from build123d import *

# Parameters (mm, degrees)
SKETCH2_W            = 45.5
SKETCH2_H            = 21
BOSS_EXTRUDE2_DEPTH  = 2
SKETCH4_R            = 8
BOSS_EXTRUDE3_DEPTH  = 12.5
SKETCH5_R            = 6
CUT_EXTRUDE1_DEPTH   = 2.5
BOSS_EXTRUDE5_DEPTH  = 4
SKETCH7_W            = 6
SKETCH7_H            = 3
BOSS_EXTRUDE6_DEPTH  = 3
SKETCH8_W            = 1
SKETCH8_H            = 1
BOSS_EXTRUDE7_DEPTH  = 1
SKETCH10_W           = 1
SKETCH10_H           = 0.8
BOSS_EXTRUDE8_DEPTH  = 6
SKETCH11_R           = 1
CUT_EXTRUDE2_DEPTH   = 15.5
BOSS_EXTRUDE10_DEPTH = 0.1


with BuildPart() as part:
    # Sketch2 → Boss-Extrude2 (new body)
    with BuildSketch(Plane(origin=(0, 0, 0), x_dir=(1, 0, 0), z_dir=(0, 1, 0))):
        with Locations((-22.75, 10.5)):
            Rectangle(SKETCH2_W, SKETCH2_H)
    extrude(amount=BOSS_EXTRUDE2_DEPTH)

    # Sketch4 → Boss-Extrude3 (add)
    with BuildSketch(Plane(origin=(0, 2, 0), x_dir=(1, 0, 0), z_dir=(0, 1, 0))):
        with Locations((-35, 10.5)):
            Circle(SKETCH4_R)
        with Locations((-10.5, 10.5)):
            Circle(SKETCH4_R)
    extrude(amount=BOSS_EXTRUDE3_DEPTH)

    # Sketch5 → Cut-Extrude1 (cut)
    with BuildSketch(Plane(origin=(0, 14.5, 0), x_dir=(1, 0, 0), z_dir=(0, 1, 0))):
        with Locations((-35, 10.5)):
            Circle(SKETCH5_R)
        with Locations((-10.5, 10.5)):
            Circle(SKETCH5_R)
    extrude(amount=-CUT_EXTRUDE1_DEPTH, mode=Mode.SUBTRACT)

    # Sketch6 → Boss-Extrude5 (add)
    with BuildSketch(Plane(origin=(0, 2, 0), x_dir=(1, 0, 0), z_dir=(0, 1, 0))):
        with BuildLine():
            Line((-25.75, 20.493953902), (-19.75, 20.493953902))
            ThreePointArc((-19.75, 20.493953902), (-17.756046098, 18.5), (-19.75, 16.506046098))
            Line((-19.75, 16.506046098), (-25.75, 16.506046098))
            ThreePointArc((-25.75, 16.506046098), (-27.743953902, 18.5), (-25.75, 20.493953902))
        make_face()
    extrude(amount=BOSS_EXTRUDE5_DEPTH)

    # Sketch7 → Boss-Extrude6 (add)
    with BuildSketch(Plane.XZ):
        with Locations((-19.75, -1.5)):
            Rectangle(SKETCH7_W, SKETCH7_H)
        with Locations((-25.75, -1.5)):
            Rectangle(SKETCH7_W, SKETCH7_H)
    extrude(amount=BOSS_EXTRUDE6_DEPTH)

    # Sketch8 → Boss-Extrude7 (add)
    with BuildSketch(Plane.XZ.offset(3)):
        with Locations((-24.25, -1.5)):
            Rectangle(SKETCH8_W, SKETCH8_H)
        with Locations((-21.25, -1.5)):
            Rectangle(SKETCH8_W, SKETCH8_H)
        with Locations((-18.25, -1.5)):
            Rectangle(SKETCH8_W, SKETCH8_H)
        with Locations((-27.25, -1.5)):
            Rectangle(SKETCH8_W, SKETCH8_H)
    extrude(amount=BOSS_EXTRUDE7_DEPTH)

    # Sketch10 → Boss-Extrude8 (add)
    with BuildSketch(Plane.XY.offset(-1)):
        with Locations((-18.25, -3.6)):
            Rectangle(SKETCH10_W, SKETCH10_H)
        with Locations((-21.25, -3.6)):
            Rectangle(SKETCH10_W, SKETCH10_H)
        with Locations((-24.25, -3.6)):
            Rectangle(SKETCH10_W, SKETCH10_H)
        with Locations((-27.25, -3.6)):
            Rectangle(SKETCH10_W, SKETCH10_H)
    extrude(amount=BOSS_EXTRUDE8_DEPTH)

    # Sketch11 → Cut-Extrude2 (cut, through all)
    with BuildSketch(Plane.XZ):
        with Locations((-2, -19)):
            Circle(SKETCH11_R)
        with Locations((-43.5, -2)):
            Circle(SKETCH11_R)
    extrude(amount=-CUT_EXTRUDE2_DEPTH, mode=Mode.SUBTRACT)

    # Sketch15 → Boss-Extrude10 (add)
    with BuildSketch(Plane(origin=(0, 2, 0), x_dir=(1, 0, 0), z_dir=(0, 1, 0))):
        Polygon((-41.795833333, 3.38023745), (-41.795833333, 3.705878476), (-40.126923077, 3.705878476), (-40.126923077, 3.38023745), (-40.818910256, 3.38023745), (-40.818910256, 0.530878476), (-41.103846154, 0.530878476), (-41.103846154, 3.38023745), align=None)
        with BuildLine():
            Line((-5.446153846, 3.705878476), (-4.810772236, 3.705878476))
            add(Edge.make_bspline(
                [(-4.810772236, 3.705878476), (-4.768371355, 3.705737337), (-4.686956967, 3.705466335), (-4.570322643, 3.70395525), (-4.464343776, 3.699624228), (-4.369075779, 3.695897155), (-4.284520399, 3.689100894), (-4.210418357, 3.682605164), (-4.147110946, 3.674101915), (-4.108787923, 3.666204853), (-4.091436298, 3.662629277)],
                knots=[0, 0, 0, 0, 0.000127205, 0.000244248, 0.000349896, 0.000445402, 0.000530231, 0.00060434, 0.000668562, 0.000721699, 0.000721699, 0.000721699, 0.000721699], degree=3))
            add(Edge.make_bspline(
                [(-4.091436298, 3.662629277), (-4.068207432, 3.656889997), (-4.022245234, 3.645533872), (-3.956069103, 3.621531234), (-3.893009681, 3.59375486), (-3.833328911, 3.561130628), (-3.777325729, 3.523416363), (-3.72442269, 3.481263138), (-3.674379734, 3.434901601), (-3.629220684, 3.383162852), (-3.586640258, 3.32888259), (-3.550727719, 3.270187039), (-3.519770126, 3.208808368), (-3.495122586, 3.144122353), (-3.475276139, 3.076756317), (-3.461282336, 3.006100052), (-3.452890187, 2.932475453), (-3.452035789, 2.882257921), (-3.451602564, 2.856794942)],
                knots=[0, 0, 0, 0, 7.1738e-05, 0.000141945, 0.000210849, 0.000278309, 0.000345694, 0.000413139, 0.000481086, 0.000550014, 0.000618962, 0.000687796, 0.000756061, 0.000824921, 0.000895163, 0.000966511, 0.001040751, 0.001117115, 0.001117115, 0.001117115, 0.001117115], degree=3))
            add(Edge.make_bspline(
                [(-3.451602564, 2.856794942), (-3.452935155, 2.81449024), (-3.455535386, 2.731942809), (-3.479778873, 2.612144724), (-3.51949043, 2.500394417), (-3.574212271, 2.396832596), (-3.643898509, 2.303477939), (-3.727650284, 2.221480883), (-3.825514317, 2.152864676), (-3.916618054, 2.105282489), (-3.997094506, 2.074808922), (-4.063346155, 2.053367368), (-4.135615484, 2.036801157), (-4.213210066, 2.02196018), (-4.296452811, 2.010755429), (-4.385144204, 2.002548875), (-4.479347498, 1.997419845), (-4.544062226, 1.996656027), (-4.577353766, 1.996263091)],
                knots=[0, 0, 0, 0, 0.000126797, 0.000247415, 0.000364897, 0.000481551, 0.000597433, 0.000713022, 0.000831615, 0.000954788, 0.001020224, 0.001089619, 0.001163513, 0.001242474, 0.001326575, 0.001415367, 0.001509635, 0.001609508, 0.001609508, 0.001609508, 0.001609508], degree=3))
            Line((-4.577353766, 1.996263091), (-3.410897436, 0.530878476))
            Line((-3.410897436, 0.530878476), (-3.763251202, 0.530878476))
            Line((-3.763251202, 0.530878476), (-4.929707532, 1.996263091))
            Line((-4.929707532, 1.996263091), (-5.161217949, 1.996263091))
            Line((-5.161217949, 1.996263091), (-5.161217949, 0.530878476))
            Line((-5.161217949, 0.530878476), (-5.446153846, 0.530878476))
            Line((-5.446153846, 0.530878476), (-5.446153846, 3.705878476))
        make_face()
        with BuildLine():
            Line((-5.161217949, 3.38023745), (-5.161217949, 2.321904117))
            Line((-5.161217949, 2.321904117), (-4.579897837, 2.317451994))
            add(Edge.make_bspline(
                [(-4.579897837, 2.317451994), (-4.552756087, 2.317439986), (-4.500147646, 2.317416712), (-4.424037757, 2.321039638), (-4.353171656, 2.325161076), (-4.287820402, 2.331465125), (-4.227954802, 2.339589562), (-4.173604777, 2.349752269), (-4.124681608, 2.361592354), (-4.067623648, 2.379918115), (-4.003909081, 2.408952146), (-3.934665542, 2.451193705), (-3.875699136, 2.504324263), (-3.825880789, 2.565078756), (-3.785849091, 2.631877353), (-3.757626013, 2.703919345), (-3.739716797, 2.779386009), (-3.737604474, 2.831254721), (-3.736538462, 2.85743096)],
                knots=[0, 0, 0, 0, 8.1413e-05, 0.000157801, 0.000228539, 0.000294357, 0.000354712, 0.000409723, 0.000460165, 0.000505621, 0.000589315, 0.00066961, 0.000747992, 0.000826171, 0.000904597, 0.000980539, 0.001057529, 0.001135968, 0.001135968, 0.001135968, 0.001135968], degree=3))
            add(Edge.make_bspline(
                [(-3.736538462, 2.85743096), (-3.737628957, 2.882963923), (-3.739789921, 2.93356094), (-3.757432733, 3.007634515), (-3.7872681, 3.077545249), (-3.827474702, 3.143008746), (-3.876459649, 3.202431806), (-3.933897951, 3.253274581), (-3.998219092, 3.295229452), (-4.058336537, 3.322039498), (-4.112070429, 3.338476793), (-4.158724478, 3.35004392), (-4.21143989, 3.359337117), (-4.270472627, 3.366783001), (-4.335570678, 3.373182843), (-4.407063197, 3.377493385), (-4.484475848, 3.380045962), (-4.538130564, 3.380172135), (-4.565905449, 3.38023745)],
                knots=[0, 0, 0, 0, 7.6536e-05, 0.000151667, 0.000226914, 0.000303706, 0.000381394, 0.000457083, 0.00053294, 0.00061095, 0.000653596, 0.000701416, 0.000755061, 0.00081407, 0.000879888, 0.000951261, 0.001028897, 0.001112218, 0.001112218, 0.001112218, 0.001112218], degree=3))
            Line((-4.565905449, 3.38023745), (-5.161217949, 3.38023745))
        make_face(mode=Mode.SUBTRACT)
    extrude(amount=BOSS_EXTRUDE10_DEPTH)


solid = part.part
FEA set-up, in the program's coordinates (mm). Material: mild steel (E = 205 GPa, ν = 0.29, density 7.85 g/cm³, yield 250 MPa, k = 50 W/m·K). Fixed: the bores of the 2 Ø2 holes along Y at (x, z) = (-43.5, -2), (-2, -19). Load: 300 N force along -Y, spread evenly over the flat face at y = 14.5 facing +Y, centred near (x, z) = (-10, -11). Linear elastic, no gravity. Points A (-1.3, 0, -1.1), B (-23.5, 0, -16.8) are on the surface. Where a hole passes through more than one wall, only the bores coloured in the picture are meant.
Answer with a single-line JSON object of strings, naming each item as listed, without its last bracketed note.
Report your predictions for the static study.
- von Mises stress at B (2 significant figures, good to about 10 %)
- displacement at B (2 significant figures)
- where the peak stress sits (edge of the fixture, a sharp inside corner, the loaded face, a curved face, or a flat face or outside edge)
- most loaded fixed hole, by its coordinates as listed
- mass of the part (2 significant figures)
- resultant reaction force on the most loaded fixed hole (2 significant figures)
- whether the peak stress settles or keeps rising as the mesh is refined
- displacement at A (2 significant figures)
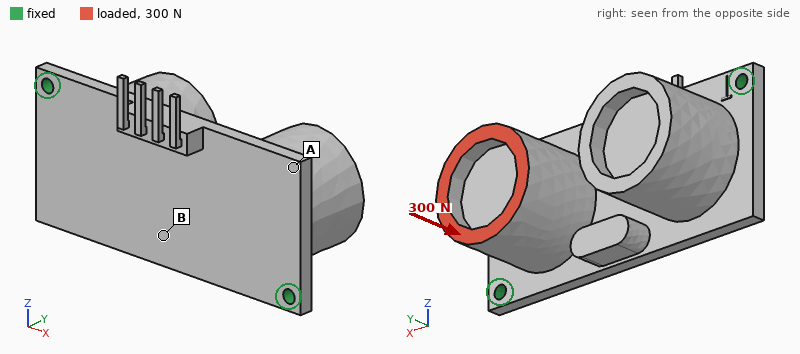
{"von Mises stress at B": "27 MPa", "displacement at B": "11 µm", "where the peak stress sits": "edge of the fixture", "most loaded fixed hole, by its coordinates as listed": "(-2, -19)", "mass of the part": "52 g", "resultant reaction force on the most loaded fixed hole": "240 N", "whether the peak stress settles or keeps rising as the mesh is refined": "keeps rising", "displacement at A": "39 µm"}
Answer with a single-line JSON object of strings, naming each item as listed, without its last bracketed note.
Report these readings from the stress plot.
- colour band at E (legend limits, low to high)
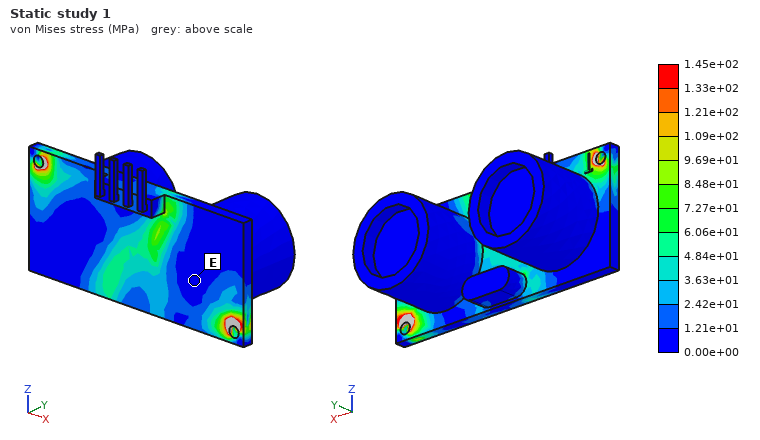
{"colour band at E": "0.00e+00 to 1.21e+01 MPa"}
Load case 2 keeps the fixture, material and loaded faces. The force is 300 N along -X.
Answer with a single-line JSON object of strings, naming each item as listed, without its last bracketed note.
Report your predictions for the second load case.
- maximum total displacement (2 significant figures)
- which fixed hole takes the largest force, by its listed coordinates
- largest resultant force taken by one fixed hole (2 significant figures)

{"maximum total displacement": "52 µm", "which fixed hole takes the largest force, by its listed coordinates": "(-2, -19)", "largest resultant force taken by one fixed hole": "190 N"}
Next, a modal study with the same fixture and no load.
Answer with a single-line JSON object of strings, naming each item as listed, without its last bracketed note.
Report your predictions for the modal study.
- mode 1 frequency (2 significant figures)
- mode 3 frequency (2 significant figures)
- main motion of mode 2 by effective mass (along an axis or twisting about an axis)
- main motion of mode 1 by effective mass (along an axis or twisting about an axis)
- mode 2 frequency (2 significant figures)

{"mode 1 frequency": "2200 Hz", "mode 3 frequency": "4900 Hz", "main motion of mode 2 by effective mass": "along Y", "main motion of mode 1 by effective mass": "along Z", "mode 2 frequency": "2600 Hz"}
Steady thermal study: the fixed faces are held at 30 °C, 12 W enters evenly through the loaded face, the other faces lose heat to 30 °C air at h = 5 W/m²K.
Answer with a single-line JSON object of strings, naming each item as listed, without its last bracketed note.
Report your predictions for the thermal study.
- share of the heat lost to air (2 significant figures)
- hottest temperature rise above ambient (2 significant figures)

{"share of the heat lost to air": "6.6 %", "hottest temperature rise above ambient": "75 K"}
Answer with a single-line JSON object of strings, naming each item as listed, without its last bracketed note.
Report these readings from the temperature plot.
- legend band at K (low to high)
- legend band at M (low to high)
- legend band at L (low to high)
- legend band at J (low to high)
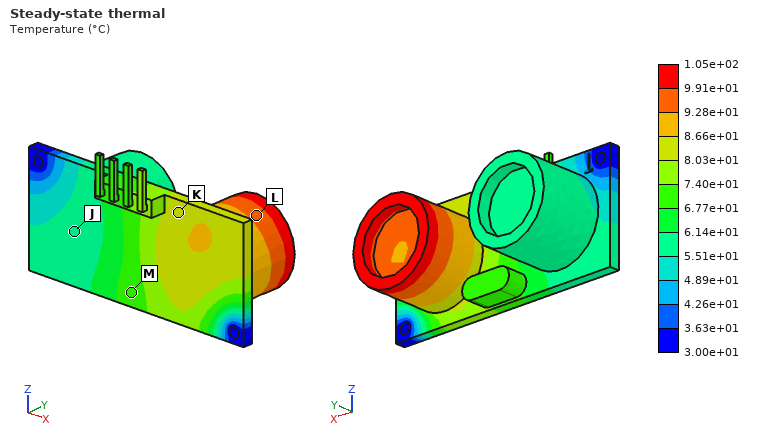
{"legend band at K": "8.03e+01 to 8.66e+01 °C", "legend band at M": "6.77e+01 to 7.40e+01 °C", "legend band at L": "9.28e+01 to 9.91e+01 °C", "legend band at J": "5.51e+01 to 6.14e+01 °C"}
